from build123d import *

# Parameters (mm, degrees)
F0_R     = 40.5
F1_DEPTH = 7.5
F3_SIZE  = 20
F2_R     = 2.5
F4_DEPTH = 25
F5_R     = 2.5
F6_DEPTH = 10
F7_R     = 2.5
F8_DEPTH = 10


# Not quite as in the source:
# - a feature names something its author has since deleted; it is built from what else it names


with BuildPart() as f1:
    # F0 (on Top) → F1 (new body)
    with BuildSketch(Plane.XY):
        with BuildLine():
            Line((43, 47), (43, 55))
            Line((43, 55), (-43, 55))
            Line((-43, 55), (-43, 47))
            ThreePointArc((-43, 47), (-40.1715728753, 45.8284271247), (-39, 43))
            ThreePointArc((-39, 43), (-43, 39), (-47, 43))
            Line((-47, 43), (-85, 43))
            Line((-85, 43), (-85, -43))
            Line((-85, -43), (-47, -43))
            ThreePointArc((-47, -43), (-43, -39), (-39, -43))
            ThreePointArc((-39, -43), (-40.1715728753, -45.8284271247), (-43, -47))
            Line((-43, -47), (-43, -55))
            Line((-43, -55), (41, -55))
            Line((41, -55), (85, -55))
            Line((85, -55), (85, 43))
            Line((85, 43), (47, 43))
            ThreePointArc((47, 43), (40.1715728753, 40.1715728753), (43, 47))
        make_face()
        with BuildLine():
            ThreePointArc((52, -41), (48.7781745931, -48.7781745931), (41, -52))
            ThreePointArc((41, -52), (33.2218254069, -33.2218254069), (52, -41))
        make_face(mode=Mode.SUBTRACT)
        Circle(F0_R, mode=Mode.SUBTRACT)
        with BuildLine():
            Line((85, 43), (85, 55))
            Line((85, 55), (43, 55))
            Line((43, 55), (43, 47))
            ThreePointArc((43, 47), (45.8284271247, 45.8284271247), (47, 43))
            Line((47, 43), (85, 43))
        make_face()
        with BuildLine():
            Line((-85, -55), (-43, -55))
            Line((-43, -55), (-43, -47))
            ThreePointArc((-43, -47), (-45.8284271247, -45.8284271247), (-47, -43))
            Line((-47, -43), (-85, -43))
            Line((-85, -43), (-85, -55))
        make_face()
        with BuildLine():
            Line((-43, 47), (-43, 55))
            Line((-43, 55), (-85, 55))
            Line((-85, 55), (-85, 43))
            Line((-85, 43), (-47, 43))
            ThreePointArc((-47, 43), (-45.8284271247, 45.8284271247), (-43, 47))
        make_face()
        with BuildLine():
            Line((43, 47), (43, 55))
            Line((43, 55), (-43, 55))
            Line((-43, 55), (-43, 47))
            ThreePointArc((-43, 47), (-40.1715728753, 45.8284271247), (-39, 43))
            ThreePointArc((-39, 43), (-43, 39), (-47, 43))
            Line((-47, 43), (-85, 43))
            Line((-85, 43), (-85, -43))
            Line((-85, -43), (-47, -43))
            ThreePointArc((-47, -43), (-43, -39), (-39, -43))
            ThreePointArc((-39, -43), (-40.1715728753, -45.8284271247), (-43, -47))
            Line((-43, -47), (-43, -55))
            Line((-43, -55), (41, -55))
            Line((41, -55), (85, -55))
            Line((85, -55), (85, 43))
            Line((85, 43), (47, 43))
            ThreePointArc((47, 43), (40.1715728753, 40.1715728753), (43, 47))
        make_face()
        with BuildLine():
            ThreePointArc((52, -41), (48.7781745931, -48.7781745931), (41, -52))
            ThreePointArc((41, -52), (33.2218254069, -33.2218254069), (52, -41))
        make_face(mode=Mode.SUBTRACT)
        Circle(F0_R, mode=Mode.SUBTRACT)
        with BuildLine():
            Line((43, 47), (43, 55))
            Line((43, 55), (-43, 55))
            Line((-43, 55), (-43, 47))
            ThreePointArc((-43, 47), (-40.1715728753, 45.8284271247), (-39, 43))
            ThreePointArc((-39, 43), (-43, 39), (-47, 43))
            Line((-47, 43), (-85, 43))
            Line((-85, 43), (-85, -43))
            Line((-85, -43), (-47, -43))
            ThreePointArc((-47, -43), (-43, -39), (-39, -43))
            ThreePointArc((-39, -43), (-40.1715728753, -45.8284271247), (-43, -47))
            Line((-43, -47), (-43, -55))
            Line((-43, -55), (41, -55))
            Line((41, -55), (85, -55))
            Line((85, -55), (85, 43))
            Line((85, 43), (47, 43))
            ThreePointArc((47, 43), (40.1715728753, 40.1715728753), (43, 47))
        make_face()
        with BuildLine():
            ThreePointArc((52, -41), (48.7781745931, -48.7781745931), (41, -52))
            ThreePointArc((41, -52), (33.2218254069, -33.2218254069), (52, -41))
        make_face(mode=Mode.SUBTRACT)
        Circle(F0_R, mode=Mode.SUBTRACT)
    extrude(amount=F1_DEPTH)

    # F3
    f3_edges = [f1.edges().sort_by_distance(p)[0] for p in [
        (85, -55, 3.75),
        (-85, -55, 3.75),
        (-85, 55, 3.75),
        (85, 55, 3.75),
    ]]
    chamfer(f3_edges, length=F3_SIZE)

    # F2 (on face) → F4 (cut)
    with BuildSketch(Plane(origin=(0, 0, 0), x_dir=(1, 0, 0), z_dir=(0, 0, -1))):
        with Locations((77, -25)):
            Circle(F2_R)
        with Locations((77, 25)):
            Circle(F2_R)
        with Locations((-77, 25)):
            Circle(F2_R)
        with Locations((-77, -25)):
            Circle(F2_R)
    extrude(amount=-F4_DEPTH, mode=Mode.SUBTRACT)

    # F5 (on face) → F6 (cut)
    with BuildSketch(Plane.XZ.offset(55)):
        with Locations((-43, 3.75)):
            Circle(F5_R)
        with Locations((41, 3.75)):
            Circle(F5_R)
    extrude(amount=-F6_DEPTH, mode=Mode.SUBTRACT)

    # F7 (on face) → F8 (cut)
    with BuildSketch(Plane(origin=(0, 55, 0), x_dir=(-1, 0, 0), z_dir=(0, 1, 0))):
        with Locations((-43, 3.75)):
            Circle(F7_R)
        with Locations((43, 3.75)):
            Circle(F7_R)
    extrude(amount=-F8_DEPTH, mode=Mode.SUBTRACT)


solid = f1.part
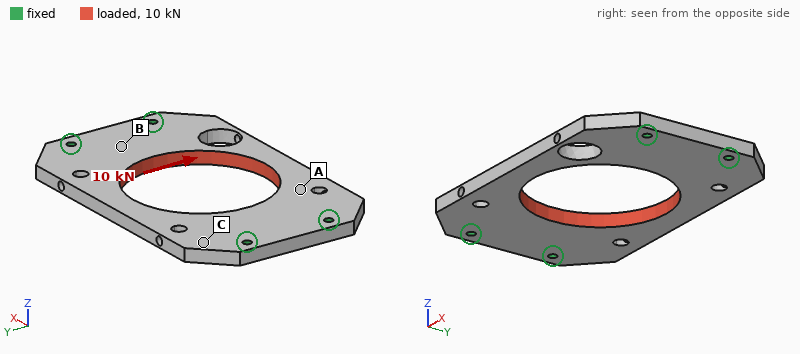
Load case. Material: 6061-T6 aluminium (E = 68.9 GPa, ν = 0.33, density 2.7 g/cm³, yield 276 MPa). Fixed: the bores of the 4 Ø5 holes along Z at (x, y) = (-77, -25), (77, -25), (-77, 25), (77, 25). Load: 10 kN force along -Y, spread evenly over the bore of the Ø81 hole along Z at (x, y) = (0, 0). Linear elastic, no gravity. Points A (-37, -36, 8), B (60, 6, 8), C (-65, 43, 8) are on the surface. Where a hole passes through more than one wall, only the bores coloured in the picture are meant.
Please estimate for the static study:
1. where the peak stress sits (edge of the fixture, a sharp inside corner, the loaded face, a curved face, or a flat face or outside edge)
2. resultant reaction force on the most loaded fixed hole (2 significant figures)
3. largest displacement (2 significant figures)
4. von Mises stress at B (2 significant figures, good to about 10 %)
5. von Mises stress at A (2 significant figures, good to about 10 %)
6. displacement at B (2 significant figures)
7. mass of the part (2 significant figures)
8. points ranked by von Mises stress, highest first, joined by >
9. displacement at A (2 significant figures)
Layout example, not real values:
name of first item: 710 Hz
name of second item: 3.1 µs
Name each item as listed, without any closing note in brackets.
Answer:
where the peak stress sits: a curved face
resultant reaction force on the most loaded fixed hole: 2.9 kN
largest displacement: 42 µm
von Mises stress at B: 23 MPa
von Mises stress at A: 12 MPa
displacement at B: 9.5 µm
mass of the part: 240 g
points ranked by von Mises stress, highest first, joined by >: B > A > C
displacement at A: 22 µm
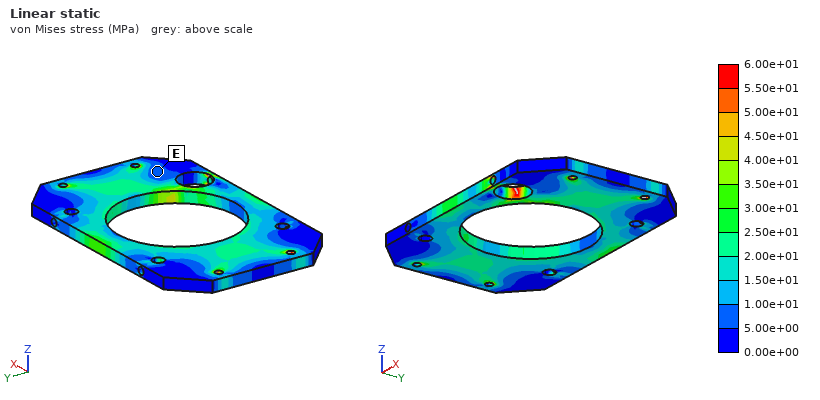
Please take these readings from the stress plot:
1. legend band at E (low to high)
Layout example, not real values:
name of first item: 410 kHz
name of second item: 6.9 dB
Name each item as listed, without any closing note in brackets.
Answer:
legend band at E: 5.00e+00 to 1.00e+01 MPa
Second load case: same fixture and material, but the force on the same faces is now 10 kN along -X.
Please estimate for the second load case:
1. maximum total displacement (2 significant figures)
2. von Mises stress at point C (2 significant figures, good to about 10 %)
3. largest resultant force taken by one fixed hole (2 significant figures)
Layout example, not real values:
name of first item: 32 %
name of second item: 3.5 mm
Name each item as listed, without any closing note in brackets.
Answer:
maximum total displacement: 20 µm
von Mises stress at point C: 4.6 MPa
largest resultant force taken by one fixed hole: 2.9 kN
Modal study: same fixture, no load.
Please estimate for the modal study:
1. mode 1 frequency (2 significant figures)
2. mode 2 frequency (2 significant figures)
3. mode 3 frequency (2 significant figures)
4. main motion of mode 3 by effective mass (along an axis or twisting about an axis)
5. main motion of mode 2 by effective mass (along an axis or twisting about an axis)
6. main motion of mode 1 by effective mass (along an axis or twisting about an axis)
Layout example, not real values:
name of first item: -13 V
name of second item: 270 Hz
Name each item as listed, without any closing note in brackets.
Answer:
mode 1 frequency: 1700 Hz
mode 2 frequency: 1800 Hz
mode 3 frequency: 3500 Hz
main motion of mode 3 by effective mass: twisting about Y
main motion of mode 2 by effective mass: twisting about X
main motion of mode 1 by effective mass: along Z
